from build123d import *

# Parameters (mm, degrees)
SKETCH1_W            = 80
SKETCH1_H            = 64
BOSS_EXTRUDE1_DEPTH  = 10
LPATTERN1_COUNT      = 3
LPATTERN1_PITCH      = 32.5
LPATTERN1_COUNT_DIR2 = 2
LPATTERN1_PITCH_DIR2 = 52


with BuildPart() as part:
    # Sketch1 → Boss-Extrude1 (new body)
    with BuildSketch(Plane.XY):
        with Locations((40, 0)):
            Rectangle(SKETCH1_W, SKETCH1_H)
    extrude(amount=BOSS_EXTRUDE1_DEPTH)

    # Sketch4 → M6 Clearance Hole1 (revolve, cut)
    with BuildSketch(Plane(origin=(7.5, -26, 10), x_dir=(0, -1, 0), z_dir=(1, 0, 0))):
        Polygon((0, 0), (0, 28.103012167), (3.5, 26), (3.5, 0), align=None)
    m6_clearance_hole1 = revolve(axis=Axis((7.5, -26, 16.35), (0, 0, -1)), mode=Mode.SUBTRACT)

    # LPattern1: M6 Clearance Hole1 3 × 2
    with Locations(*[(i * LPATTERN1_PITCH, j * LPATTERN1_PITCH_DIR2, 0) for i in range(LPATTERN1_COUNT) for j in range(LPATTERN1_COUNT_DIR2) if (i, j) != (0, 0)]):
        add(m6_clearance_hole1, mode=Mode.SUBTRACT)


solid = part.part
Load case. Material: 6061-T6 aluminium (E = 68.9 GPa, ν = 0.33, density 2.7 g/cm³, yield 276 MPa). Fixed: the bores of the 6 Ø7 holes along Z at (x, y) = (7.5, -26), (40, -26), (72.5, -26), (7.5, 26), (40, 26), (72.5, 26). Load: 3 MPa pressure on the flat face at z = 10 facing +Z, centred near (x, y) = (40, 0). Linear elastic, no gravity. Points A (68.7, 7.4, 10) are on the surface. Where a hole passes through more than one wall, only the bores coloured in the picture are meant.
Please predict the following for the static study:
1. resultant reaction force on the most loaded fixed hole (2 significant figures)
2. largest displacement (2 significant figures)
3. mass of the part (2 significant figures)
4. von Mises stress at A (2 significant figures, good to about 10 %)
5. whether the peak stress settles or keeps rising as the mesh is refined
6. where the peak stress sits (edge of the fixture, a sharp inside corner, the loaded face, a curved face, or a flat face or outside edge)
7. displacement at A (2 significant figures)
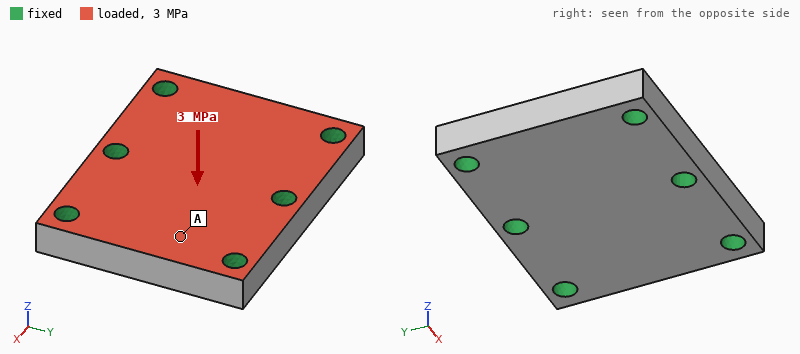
3.0 kN
15 µm
130 g
13 MPa
keeps rising
edge of the fixture
12 µm
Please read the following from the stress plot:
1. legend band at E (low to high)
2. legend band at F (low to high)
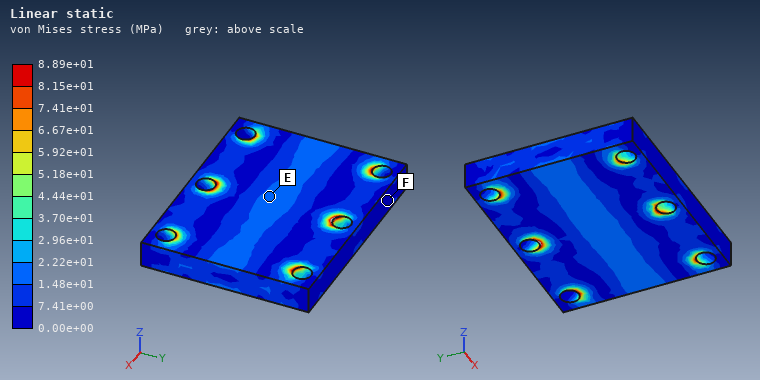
1.48e+01 to 2.22e+01 MPa
0.00e+00 to 7.41e+00 MPa
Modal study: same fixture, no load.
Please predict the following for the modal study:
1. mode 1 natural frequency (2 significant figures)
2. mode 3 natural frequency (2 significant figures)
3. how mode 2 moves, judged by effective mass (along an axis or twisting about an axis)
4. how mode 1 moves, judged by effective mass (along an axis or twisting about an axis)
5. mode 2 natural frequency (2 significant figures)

15 kHz
22 kHz
twisting about Y
along Z
18 kHz
